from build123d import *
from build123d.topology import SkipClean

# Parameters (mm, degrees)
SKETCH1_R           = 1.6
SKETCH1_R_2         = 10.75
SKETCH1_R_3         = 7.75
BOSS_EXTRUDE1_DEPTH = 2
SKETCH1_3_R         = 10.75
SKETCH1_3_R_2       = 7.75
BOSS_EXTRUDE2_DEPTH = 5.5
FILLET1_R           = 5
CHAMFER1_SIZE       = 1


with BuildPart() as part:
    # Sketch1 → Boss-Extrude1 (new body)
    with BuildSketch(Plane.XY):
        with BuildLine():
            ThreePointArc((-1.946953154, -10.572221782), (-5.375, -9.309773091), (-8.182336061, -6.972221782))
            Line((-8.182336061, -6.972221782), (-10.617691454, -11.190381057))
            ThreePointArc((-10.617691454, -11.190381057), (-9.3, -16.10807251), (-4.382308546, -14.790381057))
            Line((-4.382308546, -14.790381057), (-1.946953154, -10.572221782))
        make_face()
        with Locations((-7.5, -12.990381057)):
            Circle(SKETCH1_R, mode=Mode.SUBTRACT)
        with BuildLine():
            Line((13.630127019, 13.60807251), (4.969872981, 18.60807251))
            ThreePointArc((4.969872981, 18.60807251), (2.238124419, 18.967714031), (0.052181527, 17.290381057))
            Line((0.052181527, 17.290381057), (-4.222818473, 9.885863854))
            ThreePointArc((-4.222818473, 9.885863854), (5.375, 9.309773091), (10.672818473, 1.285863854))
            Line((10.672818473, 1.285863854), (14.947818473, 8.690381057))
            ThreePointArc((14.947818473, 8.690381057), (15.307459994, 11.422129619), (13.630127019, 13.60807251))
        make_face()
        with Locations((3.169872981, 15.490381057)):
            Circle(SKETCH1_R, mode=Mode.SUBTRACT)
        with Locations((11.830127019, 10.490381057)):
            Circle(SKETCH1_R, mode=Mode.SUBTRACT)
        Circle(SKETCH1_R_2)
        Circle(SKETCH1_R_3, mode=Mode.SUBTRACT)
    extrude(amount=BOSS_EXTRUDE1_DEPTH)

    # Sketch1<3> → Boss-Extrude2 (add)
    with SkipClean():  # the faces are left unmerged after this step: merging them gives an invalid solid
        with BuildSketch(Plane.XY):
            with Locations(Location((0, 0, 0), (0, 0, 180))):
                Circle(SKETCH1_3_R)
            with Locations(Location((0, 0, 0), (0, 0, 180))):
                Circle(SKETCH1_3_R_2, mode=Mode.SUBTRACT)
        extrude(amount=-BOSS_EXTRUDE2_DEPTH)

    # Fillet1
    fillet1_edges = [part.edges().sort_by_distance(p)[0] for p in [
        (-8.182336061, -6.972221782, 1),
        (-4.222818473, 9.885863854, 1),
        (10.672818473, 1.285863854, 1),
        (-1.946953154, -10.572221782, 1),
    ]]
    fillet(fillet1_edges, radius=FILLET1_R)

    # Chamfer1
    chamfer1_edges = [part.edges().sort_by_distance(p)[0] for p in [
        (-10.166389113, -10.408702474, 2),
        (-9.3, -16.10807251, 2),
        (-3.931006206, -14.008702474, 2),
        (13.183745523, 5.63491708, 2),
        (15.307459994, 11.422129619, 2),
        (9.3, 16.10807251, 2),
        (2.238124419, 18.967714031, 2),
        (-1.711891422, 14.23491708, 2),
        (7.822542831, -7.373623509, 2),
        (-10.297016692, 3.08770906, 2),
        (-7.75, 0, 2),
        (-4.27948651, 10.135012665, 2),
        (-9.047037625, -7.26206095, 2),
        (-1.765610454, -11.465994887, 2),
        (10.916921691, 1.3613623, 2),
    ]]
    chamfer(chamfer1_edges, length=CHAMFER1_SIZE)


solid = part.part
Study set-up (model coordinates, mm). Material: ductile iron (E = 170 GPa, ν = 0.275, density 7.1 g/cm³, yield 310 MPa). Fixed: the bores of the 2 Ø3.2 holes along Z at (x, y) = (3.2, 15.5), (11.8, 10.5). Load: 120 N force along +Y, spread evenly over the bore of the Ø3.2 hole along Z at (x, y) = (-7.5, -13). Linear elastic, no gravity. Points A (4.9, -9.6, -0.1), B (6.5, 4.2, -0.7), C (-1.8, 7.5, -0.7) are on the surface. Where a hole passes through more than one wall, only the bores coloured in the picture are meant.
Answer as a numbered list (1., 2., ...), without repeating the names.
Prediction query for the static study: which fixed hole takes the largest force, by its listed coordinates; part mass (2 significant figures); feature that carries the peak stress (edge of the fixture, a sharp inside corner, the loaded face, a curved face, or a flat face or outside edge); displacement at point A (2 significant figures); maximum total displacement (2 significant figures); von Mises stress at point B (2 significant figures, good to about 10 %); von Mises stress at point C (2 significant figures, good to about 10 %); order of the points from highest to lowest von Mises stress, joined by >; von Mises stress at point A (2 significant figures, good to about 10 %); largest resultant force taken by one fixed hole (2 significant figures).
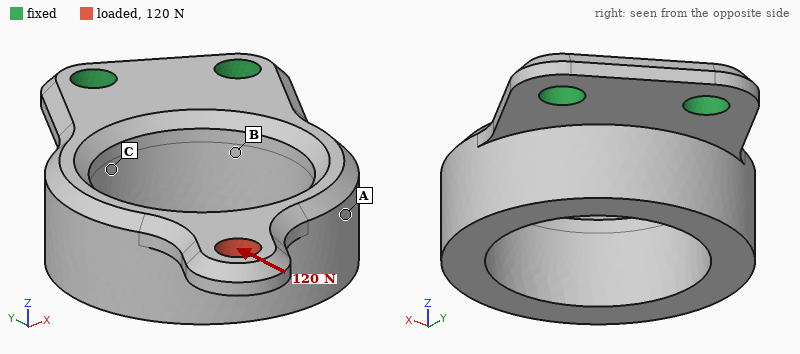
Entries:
1. (3.2, 15.5)
2. 11 g
3. a curved face
4. 9.3 µm
5. 16 µm
6. 17 MPa
7. 33 MPa
8. C > B > A
9. 7.8 MPa
10. 200 N
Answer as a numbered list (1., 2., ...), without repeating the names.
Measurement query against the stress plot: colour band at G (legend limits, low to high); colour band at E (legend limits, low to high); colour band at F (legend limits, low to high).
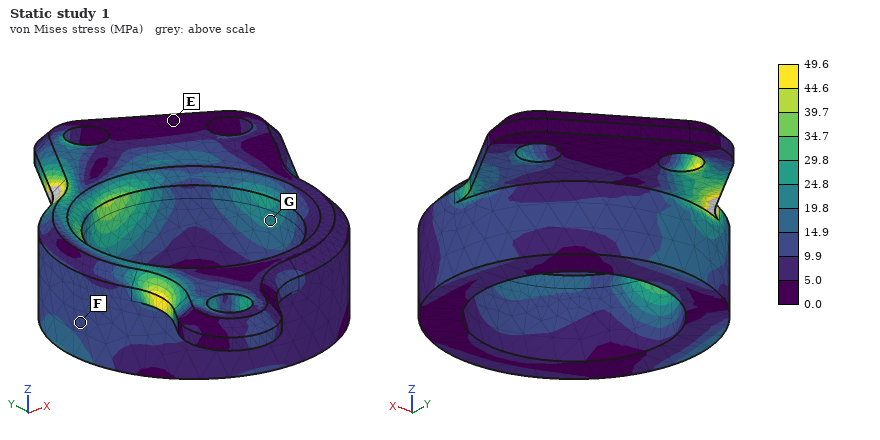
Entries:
1. 19.8 to 24.8 MPa
2. 0.0 to 5.0 MPa
3. 9.9 to 14.9 MPa
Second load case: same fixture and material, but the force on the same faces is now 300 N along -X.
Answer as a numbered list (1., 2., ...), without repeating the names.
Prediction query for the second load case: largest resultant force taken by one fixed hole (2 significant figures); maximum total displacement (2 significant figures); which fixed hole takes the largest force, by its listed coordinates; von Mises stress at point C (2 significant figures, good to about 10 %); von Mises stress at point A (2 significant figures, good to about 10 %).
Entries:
1. 720 N
2. 61 µm
3. (11.8, 10.5)
4. 110 MPa
5. 38 MPa
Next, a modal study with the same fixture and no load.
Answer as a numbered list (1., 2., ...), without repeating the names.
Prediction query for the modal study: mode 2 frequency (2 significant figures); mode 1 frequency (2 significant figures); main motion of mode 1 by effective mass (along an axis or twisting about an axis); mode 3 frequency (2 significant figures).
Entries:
1. 6100 Hz
2. 2000 Hz
3. along Z
4. 8300 Hz
